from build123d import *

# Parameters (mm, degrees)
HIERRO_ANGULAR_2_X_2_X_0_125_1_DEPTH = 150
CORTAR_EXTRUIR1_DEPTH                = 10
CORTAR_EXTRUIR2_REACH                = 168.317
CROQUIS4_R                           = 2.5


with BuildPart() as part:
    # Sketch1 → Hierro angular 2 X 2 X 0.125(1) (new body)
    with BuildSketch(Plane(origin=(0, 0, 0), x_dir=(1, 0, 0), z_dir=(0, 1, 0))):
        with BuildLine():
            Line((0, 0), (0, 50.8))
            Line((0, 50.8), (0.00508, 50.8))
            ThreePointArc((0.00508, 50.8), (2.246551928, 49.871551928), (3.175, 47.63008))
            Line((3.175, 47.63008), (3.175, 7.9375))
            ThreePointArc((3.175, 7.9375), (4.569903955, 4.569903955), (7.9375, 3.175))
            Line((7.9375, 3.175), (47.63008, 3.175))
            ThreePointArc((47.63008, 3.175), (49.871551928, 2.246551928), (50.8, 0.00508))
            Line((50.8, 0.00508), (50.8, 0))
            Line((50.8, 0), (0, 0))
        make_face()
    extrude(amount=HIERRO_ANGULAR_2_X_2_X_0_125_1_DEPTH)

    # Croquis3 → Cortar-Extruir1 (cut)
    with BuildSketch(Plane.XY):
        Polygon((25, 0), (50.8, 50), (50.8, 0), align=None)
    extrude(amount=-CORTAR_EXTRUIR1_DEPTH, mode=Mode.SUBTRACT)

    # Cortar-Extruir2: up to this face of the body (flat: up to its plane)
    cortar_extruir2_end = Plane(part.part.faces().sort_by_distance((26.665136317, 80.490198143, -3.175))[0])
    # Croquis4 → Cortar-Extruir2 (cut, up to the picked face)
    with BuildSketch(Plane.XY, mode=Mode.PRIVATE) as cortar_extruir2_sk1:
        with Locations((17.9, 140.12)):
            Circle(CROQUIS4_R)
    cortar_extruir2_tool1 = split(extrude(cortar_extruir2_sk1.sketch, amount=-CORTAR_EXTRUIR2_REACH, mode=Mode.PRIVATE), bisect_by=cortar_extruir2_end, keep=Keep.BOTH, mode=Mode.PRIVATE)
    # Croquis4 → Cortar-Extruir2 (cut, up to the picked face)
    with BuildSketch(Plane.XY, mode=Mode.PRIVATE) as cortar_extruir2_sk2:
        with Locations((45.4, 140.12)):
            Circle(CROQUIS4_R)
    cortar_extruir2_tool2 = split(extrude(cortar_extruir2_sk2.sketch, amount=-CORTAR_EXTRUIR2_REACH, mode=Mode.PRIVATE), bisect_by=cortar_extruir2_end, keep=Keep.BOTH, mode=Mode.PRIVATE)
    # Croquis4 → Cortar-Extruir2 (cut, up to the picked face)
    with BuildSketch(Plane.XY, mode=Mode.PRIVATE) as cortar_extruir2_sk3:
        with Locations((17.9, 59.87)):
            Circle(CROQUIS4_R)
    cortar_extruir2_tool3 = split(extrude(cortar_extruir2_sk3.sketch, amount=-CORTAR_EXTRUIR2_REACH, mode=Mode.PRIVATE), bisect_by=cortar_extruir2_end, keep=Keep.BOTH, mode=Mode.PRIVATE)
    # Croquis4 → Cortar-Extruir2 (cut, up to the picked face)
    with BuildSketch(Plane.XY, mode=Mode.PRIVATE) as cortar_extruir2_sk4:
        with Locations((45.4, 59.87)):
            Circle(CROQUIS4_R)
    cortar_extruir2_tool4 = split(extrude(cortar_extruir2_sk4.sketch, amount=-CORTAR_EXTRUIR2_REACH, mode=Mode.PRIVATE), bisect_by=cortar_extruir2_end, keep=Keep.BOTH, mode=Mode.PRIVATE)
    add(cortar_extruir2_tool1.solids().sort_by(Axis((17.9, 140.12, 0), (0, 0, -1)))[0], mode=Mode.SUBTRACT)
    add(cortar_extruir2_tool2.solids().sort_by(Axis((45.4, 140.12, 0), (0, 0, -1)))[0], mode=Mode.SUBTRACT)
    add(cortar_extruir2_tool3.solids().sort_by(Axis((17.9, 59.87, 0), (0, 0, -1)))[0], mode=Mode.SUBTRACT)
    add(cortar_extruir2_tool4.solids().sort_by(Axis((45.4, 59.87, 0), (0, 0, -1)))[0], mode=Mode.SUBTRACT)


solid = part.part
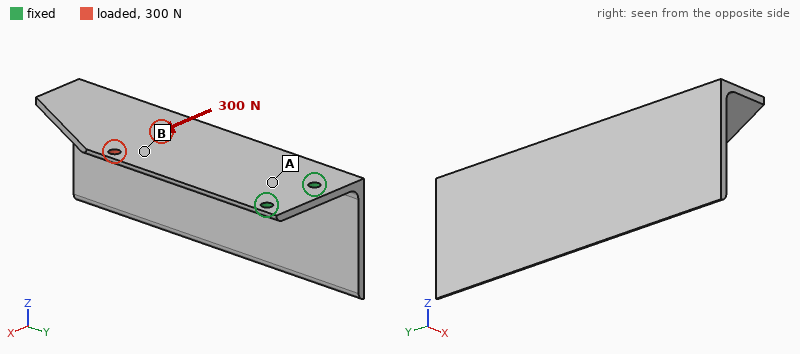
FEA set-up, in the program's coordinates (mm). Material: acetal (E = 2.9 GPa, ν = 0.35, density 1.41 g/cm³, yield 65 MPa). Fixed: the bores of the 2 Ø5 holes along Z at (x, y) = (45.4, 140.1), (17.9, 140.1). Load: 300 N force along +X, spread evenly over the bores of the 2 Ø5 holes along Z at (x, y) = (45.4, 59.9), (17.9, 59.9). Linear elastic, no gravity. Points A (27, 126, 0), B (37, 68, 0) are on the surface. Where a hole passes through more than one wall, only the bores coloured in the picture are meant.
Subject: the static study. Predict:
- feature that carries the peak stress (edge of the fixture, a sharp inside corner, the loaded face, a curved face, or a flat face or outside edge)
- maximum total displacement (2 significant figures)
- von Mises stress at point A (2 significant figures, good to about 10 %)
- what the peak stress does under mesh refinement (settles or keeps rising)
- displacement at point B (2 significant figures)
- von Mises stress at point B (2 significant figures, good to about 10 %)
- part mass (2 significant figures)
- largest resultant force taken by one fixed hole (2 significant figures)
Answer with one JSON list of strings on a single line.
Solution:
["edge of the fixture", "1.7 mm", "8.5 MPa", "keeps rising", "0.82 mm", "4.2 MPa", "63 g", "820 N"]
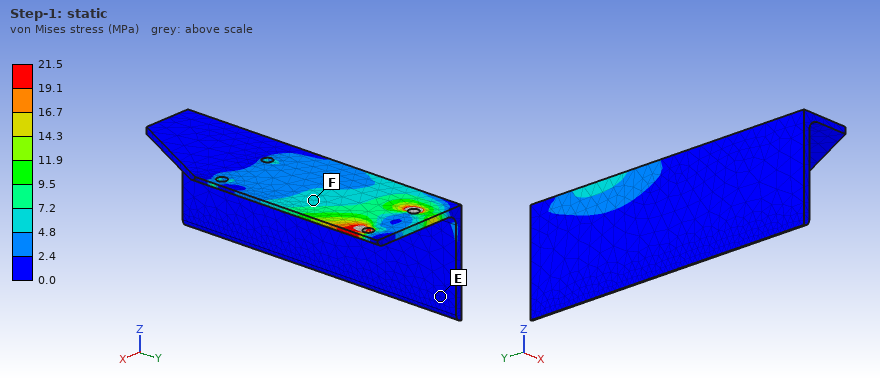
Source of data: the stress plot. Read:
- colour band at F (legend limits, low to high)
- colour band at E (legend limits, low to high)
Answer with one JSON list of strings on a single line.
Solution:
["4.8 to 7.2 MPa", "0.0 to 2.4 MPa"]
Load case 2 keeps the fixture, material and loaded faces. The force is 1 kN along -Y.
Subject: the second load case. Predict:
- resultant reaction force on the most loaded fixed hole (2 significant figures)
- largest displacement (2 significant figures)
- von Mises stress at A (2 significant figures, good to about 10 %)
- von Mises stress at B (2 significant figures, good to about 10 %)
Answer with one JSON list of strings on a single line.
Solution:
["510 N", "0.57 mm", "6.0 MPa", "7.1 MPa"]
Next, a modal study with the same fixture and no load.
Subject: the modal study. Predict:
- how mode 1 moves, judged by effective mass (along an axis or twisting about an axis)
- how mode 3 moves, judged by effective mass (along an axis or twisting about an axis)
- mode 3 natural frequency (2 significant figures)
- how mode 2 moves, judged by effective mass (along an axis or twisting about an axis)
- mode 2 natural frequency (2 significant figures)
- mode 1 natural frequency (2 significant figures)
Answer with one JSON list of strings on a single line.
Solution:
["along Z", "twisting about Z", "280 Hz", "along X", "120 Hz", "51 Hz"]
